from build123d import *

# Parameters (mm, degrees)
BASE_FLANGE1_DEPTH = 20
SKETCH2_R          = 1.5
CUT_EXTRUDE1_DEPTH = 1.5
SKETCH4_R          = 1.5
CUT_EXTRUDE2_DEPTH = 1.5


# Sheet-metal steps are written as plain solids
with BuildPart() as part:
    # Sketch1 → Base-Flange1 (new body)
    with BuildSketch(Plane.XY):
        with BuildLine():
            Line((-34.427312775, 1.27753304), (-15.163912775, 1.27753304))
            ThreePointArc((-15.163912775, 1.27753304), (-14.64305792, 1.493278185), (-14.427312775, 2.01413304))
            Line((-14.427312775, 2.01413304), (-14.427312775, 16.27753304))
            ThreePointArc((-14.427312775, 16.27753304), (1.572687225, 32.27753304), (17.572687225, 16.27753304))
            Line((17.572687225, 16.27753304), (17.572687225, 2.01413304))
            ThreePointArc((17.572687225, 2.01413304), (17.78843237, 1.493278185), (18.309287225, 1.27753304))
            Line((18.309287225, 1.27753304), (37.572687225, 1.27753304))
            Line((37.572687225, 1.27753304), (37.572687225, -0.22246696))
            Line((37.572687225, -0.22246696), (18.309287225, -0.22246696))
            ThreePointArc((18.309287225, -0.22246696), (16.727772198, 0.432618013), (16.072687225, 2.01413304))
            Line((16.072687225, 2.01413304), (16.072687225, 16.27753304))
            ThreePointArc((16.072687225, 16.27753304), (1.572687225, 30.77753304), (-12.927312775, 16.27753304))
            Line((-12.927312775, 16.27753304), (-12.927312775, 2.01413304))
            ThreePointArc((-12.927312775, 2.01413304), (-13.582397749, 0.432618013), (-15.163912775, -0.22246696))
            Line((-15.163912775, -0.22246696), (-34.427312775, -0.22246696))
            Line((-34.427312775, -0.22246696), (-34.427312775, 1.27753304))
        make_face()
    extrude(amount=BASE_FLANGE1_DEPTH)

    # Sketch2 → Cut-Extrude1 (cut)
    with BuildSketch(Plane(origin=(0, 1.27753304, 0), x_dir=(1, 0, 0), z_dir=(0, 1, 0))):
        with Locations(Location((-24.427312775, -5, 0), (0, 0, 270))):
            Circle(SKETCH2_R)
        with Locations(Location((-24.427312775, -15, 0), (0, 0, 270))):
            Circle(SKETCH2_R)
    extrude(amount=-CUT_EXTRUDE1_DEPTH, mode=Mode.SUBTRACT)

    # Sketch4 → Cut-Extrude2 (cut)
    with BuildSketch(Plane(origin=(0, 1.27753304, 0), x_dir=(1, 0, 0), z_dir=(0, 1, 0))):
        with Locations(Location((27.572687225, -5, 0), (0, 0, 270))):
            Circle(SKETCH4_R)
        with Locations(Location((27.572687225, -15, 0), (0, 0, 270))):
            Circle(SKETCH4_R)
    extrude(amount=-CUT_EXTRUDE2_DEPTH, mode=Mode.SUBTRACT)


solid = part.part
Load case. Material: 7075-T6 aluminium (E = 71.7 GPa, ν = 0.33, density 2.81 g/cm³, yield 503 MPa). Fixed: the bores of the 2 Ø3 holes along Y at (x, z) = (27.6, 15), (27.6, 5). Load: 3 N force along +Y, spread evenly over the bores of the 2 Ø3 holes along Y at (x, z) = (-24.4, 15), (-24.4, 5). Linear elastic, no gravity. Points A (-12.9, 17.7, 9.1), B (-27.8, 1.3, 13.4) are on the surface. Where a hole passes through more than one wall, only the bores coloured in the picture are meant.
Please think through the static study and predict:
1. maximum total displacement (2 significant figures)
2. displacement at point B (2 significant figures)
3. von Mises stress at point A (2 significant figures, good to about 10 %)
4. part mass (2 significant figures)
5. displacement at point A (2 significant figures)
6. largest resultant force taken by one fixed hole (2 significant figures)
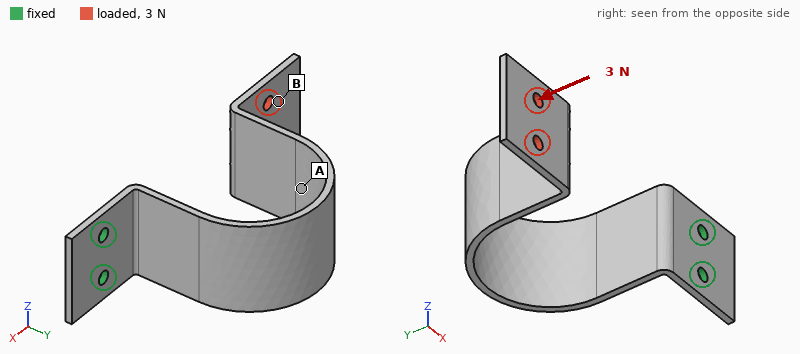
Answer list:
0.83 mm
0.71 mm
4.2 MPa
10.0 g
0.41 mm
2.2 N
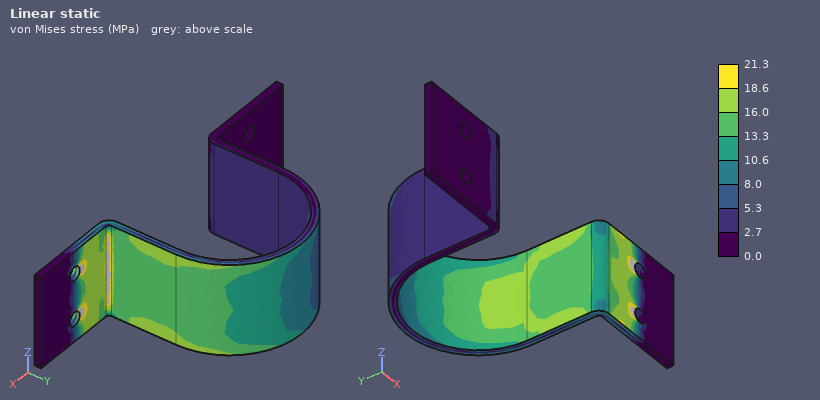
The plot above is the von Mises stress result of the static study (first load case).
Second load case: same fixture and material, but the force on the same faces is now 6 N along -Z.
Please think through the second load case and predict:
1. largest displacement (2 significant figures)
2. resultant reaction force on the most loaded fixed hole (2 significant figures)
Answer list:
0.87 mm
27 N
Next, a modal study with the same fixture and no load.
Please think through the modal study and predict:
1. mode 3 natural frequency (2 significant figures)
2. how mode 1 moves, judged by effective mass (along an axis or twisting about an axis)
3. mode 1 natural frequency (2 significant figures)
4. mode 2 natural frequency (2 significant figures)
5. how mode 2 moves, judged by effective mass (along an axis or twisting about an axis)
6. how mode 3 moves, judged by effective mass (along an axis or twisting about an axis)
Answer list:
390 Hz
along Y
180 Hz
270 Hz
along Z
along X
